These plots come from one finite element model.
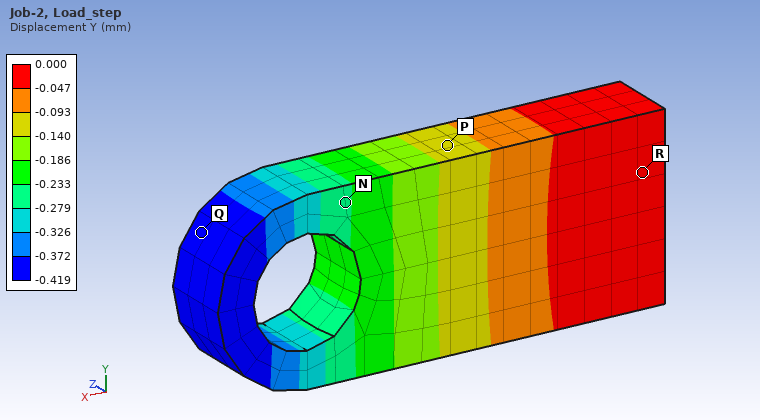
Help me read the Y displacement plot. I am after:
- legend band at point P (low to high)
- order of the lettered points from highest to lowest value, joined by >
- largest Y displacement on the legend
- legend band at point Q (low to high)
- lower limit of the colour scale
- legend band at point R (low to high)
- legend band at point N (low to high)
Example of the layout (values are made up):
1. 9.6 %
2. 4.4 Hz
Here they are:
1. -0.140 to -0.093 mm
2. R > P > N > Q
3. 0.000 mm
4. -0.419 to -0.372 mm
5. -0.419 mm
6. -0.047 to 0.000 mm
7. -0.279 to -0.233 mm
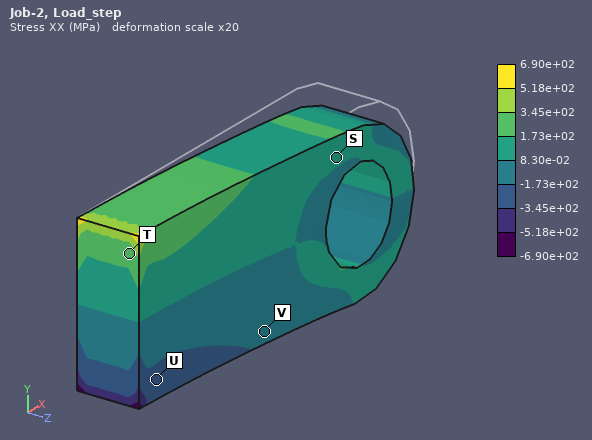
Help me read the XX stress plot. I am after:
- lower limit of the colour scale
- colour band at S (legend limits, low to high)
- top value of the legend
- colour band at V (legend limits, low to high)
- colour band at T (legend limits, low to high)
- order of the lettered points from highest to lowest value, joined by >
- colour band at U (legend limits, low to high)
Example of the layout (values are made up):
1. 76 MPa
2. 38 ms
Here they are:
1. -6.90e+02 MPa
2. 8.30e-02 to 1.73e+02 MPa
3. 6.90e+02 MPa
4. -1.73e+02 to 8.30e-02 MPa
5. 1.73e+02 to 3.45e+02 MPa
6. T > S > V > U
7. -3.45e+02 to -1.73e+02 MPa
